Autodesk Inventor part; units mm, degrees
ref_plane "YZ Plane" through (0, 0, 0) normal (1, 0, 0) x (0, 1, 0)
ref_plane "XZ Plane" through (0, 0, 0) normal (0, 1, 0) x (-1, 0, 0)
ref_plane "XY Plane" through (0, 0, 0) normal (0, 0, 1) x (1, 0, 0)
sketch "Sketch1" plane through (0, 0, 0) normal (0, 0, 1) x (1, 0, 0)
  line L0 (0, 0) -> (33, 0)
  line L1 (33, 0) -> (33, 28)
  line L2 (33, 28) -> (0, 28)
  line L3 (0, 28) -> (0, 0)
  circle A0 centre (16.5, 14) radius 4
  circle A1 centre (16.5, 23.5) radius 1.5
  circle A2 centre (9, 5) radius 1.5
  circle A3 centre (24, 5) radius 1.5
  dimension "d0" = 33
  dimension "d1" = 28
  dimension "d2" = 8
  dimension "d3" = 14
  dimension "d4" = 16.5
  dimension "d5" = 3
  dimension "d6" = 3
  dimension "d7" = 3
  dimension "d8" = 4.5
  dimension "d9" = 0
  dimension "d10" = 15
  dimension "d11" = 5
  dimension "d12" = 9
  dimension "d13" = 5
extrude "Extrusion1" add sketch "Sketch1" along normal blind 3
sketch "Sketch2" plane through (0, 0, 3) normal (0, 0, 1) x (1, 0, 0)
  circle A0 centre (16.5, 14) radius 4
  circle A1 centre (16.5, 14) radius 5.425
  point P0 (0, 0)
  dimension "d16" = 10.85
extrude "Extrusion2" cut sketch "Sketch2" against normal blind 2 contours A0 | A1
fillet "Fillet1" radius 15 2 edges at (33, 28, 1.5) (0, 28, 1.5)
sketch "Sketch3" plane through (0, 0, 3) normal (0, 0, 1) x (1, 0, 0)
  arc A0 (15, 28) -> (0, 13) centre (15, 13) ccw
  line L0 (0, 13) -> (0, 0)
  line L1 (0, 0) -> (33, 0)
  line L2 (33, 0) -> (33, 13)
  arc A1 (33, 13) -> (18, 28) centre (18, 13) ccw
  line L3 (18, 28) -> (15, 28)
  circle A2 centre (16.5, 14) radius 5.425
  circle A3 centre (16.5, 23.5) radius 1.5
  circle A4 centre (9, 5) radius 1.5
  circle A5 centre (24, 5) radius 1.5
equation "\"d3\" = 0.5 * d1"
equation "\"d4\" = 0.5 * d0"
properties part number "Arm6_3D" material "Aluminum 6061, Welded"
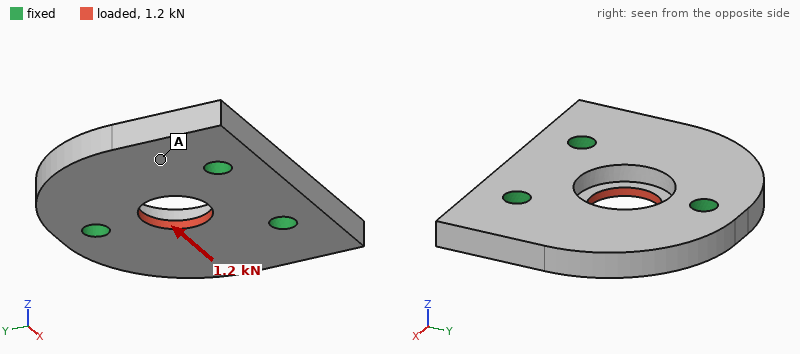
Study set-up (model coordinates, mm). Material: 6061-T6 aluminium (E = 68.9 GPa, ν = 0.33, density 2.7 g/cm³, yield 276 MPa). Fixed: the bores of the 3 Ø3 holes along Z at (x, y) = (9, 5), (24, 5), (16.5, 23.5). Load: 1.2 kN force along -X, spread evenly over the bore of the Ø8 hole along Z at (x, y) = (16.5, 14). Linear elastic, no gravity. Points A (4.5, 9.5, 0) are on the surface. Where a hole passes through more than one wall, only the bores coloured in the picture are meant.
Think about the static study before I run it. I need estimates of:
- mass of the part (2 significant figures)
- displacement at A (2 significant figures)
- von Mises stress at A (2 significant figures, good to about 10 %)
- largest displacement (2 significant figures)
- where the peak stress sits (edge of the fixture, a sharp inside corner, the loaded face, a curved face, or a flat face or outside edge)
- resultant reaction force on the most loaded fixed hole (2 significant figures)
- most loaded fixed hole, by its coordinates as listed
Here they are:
5.9 g
2.4 µm
12 MPa
6.5 µm
the loaded face
560 N
(16.5, 23.5)
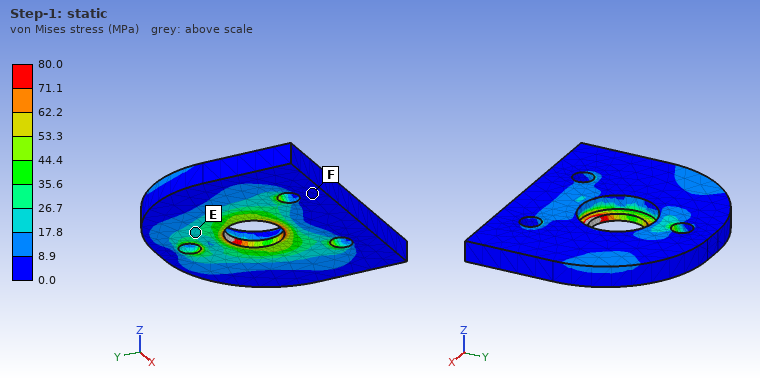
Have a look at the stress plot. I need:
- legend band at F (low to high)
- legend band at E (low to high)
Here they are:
0.0 to 8.9 MPa
17.8 to 26.7 MPa
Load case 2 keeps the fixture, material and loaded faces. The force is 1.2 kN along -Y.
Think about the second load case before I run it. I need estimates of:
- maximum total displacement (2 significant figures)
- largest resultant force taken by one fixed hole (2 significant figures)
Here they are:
5.8 µm
430 N
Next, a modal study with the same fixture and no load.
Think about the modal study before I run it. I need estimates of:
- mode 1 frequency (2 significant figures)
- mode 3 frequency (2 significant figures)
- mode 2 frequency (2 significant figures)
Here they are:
16 kHz
33 kHz
17 kHz
